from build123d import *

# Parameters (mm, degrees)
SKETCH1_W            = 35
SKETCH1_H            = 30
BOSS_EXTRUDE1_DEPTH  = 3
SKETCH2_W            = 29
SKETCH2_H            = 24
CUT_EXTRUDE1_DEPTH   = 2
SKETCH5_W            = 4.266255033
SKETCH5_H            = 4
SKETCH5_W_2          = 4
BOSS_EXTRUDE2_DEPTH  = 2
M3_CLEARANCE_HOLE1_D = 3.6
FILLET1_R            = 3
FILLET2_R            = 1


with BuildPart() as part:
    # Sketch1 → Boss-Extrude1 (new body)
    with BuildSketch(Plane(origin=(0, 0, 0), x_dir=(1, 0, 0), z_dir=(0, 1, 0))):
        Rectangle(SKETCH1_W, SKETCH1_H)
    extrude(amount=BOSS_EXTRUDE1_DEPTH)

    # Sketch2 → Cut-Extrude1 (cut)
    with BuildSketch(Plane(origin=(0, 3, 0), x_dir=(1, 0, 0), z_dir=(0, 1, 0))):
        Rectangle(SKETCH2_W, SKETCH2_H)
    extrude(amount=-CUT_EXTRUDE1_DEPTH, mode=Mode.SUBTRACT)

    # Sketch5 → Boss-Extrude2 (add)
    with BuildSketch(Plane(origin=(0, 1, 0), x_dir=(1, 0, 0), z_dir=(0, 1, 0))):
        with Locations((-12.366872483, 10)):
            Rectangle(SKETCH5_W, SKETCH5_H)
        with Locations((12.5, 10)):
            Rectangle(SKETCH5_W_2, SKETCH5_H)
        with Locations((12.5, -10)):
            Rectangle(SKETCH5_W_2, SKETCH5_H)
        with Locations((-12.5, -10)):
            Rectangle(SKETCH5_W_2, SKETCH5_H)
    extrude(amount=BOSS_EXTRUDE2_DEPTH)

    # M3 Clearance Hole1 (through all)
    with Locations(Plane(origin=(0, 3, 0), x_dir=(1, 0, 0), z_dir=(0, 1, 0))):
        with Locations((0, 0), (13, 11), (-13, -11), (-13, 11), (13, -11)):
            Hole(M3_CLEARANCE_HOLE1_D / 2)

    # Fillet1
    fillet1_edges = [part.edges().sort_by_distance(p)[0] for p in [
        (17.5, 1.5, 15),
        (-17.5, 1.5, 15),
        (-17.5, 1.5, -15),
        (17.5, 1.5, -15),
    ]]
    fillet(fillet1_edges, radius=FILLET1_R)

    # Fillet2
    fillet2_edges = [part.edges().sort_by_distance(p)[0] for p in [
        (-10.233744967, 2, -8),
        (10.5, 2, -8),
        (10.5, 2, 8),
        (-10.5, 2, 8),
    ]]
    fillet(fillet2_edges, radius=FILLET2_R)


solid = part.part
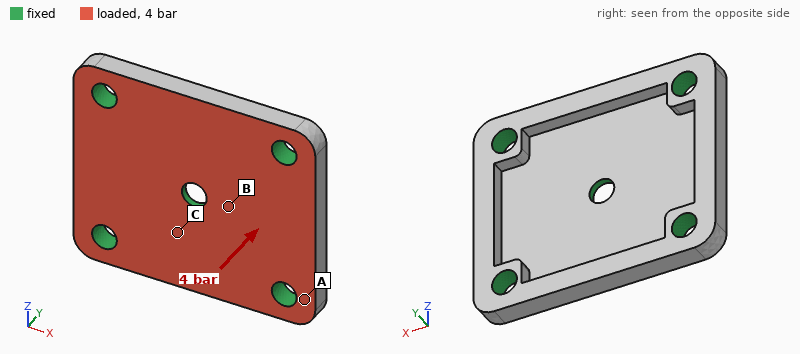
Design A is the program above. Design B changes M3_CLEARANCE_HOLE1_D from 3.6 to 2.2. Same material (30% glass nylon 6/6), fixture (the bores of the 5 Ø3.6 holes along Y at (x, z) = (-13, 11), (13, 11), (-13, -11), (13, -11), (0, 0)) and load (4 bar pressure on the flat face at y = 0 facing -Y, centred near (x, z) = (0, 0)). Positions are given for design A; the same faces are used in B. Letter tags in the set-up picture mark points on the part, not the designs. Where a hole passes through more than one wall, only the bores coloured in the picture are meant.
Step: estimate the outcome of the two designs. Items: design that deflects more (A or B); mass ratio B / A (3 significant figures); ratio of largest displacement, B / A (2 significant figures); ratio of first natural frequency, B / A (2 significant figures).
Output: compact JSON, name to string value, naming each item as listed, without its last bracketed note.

{"design that deflects more": "B", "mass ratio B / A": "1.05", "ratio of largest displacement, B / A": "1.2", "ratio of first natural frequency, B / A": "0.90"}
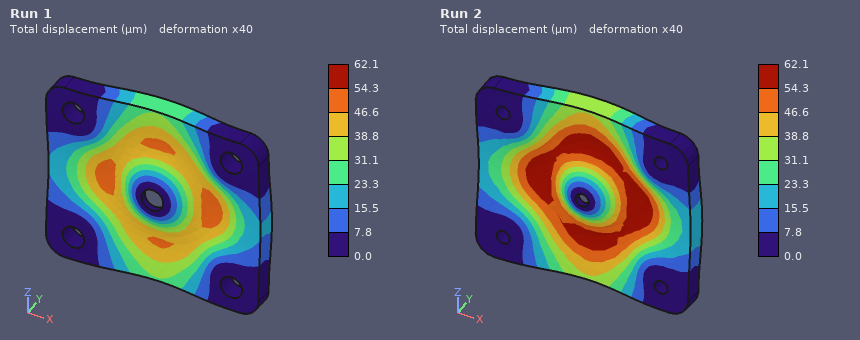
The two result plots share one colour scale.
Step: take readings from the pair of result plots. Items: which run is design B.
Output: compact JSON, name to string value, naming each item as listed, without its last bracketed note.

{"which run is design B": "Run 2"}
